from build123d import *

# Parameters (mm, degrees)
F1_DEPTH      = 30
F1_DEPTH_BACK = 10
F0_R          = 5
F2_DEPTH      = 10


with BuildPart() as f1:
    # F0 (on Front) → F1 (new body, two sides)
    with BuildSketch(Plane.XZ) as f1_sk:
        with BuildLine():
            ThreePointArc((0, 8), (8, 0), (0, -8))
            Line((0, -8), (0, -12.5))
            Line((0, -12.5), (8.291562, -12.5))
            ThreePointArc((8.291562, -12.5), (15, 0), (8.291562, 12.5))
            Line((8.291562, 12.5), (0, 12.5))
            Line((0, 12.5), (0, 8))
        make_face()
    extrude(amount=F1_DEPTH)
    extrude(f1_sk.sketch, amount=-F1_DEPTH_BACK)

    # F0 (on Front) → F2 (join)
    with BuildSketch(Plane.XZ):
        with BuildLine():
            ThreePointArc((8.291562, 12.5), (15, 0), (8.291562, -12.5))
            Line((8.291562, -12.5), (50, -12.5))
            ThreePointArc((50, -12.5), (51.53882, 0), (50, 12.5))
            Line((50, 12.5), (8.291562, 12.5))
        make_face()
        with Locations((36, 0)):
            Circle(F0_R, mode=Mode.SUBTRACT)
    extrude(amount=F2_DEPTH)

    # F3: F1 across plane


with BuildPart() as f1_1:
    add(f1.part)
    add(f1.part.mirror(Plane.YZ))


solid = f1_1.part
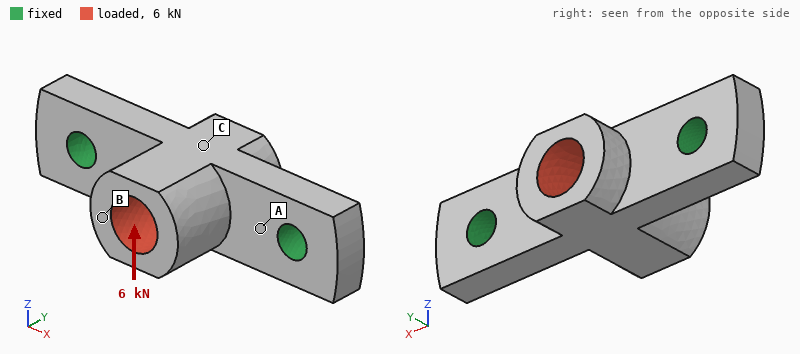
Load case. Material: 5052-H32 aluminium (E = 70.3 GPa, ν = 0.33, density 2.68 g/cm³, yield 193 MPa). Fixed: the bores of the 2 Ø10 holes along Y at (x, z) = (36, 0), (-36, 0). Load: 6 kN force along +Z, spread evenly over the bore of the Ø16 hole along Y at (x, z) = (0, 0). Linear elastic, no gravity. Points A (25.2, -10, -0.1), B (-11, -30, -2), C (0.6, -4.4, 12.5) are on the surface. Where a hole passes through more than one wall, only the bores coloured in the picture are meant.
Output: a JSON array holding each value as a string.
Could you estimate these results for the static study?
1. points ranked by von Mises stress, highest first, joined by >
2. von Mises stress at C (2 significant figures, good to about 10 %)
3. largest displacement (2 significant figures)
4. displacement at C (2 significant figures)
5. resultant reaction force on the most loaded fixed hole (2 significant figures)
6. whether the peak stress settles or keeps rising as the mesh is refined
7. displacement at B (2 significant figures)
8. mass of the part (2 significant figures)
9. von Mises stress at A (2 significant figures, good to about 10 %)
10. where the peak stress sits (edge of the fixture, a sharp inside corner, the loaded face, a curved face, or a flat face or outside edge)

["A > C > B", "36 MPa", "77 µm", "32 µm", "3.0 kN", "keeps rising", "72 µm", "95 g", "62 MPa", "edge of the fixture"]
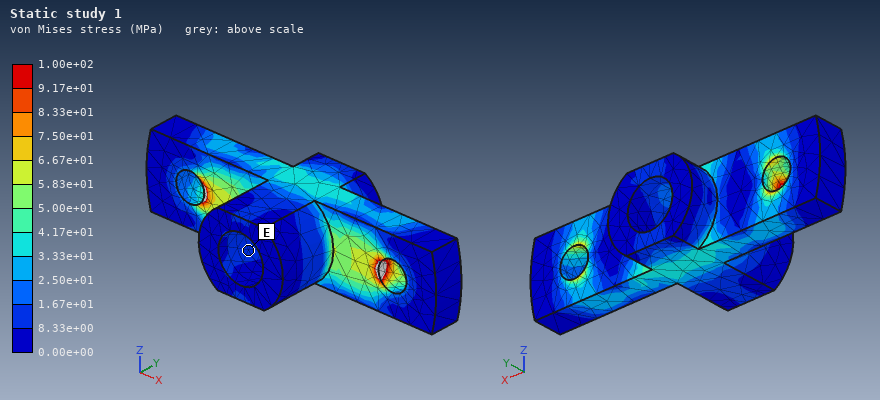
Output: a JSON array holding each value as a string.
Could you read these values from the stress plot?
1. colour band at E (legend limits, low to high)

["8.33e+00 to 1.67e+01 MPa"]
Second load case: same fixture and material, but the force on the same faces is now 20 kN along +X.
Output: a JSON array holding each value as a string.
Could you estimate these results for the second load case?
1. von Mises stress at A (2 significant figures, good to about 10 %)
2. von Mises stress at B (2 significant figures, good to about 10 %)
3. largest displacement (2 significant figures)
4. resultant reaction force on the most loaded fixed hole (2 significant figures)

["55 MPa", "21 MPa", "60 µm", "10 kN"]
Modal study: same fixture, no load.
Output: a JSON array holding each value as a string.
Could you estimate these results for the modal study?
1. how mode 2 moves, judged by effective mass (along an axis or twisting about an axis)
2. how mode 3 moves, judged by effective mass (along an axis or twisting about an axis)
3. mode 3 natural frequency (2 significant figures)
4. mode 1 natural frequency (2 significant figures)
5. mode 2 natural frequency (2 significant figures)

["along Y", "along Z", "12 kHz", "6200 Hz", "8800 Hz"]
